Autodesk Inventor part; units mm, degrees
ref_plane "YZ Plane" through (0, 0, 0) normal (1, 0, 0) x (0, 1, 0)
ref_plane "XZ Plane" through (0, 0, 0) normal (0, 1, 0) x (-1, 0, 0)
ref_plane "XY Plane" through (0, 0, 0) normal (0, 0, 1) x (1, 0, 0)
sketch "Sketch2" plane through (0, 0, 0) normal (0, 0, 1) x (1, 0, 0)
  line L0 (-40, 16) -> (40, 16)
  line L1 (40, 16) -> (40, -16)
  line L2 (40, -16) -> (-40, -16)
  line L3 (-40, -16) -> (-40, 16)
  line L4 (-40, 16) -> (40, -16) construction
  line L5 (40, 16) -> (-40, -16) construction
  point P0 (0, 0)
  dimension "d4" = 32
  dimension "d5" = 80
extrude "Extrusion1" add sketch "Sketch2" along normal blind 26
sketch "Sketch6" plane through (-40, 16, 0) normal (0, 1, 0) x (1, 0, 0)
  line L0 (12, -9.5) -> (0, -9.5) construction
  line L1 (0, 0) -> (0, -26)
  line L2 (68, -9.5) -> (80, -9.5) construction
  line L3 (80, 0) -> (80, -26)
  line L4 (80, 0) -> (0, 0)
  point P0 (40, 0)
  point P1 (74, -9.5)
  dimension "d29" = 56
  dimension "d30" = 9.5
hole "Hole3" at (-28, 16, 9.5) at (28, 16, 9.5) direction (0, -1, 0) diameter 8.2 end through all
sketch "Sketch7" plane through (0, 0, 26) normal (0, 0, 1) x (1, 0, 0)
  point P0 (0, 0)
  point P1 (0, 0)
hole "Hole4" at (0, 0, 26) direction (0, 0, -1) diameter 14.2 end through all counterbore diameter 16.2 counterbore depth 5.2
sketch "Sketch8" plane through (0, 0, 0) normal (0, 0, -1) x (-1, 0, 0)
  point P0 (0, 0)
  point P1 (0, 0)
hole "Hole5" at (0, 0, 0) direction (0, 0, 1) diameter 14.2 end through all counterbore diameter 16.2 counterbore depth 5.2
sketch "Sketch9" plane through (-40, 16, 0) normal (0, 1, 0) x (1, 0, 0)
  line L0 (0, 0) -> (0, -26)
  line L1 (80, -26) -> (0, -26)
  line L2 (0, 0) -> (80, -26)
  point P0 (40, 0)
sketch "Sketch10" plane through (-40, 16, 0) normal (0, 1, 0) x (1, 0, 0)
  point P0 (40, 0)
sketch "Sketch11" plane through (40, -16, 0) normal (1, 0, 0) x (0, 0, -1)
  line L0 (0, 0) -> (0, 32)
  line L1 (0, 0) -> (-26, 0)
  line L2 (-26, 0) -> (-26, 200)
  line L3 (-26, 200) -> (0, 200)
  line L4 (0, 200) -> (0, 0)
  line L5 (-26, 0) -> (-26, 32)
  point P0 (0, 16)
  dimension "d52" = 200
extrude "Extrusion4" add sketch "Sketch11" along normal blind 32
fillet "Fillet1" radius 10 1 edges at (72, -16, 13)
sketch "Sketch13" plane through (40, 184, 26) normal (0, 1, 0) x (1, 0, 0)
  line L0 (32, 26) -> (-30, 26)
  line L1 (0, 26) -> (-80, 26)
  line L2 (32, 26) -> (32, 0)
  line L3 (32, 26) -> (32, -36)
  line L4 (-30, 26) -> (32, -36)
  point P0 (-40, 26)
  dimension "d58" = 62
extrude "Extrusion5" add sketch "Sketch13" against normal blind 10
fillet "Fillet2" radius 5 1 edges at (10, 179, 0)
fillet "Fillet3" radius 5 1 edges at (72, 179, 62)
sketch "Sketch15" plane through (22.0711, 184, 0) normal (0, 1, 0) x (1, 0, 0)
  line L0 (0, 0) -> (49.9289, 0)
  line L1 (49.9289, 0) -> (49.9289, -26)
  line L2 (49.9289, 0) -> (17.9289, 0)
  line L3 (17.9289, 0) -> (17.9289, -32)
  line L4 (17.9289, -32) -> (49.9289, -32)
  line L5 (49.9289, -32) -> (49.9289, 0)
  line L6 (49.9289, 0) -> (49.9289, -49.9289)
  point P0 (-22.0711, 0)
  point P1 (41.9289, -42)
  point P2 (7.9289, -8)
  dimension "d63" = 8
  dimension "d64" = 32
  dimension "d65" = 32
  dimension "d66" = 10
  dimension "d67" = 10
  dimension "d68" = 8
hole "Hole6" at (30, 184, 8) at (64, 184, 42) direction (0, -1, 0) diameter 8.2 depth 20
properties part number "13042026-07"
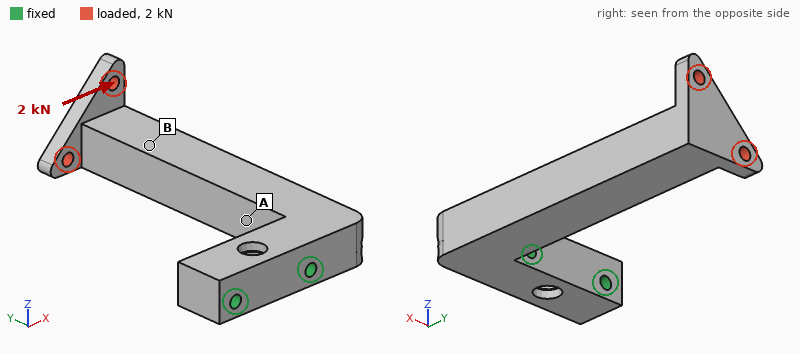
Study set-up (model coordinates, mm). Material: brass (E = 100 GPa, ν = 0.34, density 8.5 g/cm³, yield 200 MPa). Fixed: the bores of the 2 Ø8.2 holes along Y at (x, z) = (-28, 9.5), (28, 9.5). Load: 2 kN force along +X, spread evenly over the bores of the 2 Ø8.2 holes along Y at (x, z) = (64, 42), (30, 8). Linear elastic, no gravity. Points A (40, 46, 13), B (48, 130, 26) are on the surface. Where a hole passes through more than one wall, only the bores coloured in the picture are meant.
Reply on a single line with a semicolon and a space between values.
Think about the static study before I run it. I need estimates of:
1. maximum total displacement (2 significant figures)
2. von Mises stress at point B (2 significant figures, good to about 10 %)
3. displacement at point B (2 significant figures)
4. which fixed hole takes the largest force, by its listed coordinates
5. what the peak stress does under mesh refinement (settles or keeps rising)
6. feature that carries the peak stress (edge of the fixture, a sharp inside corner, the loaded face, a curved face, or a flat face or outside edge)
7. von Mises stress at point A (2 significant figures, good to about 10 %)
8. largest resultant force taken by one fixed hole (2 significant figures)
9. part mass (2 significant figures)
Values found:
0.81 mm; 17 MPa; 0.46 mm; (28, 9.5); keeps rising; edge of the fixture; 59 MPa; 1.7 kN; 2.0 kg
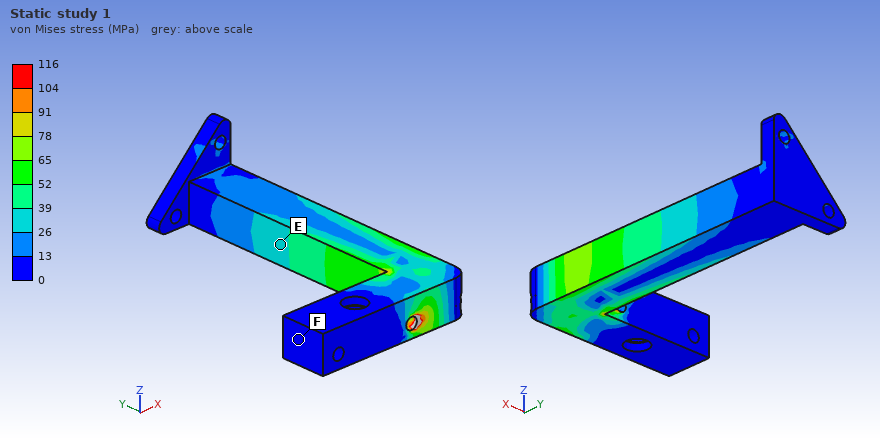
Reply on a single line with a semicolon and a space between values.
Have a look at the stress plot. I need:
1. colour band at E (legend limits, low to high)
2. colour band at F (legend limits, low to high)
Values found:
26 to 39 MPa; 0 to 13 MPa
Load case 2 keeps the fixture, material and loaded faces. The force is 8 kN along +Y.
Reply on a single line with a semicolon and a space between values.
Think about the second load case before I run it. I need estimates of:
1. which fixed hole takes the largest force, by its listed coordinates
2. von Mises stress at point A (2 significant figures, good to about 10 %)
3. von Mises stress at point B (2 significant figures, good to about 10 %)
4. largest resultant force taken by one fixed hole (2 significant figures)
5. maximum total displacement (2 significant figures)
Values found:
(28, 9.5); 26 MPa; 44 MPa; 8.1 kN; 0.55 mm
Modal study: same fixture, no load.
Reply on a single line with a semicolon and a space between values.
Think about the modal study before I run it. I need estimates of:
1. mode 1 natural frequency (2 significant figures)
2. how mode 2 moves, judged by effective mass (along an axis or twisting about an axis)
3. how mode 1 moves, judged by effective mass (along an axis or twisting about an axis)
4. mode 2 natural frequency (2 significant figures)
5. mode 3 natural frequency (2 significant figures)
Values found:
320 Hz; along X; along Z; 390 Hz; 1700 Hz
